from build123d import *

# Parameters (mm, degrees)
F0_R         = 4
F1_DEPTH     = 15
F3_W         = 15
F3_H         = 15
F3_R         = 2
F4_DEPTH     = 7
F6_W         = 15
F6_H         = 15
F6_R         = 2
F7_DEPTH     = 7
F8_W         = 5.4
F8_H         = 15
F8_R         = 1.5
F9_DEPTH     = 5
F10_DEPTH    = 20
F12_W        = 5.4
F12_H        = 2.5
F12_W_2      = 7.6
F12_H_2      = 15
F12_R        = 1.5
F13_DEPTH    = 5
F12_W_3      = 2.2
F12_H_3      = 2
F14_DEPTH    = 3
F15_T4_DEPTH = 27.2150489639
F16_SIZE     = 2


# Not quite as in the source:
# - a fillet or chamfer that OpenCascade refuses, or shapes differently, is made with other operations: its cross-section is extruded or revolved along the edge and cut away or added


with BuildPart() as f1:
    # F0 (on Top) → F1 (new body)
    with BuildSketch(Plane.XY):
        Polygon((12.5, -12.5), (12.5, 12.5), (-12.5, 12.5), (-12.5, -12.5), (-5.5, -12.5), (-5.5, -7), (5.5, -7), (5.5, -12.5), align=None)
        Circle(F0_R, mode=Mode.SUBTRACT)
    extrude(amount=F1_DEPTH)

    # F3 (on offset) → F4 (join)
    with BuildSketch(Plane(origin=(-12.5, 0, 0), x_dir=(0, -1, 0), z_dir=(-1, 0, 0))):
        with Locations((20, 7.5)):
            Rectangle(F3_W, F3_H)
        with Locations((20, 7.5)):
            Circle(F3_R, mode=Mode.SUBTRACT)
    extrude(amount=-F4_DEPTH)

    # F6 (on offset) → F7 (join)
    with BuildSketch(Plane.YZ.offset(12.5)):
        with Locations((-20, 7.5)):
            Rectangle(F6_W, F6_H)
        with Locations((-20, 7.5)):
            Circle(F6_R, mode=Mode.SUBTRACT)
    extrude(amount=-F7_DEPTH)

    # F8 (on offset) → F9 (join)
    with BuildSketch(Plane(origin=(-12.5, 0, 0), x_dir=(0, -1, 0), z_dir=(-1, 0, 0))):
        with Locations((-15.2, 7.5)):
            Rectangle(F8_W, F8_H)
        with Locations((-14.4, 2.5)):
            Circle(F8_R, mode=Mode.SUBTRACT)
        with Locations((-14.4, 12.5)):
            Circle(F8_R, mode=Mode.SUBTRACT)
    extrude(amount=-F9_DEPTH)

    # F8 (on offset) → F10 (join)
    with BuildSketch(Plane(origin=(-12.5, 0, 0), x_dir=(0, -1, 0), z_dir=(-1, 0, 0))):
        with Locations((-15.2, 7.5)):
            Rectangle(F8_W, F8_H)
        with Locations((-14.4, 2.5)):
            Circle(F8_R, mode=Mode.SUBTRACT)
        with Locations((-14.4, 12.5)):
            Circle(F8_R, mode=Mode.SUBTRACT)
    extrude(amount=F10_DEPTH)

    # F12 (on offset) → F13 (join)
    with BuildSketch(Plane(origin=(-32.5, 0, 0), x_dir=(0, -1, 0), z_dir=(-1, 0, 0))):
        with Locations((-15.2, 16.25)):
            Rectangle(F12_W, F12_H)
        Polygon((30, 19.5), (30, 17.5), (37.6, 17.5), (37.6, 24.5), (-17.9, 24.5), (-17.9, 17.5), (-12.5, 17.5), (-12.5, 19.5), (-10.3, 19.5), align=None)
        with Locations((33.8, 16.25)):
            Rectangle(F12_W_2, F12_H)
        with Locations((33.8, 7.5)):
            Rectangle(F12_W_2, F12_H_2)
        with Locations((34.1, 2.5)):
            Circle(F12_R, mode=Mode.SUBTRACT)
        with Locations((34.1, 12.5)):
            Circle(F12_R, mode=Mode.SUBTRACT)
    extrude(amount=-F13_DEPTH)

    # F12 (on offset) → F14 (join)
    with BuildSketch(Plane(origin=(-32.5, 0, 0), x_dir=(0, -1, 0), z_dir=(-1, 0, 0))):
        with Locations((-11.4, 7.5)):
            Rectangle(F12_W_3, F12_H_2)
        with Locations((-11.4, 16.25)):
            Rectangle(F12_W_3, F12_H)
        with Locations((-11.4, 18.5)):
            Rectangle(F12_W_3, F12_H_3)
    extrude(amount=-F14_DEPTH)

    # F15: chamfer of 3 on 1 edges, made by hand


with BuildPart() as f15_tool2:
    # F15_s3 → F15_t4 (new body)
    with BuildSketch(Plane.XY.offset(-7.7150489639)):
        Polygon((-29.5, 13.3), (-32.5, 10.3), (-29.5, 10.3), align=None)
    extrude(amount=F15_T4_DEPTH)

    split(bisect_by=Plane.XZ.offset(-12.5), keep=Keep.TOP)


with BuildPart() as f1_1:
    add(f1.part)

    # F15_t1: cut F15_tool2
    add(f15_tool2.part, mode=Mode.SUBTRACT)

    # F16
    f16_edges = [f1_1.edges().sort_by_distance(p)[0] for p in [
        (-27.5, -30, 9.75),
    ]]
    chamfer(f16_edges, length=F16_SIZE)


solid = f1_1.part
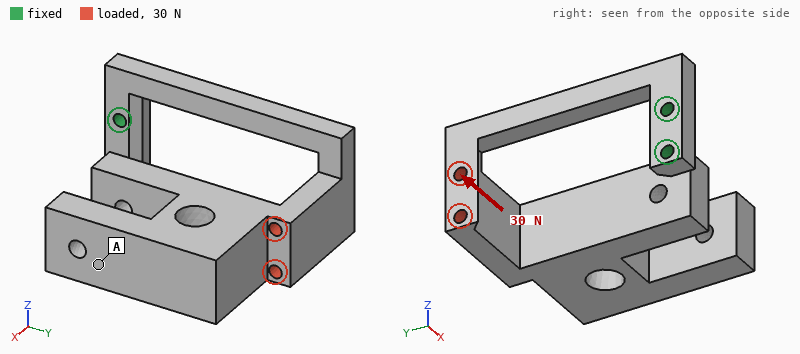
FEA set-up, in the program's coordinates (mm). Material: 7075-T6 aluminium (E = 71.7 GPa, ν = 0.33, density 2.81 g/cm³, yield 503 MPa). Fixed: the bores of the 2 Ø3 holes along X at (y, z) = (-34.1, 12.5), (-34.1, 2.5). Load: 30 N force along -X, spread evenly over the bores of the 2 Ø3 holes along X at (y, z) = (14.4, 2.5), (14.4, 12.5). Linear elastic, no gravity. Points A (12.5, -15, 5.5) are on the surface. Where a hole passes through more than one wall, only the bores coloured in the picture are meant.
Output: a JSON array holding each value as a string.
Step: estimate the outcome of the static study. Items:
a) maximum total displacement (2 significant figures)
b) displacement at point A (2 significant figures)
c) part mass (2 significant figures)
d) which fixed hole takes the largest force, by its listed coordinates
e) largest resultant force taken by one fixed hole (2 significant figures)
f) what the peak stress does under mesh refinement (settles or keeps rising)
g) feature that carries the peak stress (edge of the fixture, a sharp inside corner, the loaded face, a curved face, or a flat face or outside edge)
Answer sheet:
["0.82 mm", "0.64 mm", "41 g", "(-34.1, 12.5)", "30 N", "keeps rising", "edge of the fixture"]
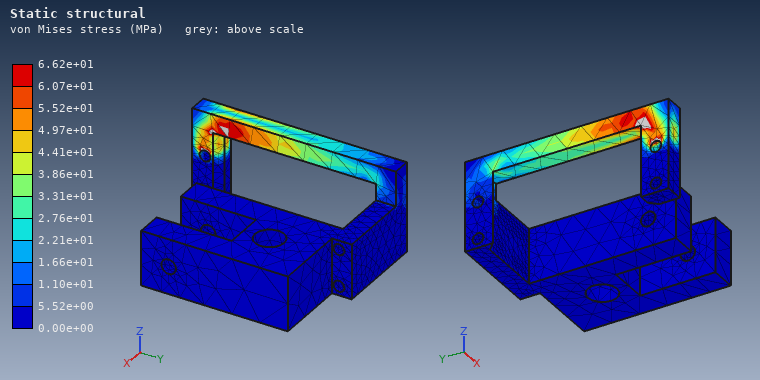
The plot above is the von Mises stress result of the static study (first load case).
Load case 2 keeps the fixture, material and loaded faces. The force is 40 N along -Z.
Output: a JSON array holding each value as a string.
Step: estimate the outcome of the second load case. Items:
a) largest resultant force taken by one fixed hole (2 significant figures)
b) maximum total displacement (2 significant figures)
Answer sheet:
["69 N", "0.89 mm"]
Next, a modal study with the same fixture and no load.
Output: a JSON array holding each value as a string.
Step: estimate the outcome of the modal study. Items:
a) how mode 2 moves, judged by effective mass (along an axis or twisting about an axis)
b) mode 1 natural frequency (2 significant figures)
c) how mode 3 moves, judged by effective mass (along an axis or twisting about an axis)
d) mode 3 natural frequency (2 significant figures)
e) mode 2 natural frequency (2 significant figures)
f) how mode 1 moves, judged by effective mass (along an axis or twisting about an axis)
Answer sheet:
["along Y", "160 Hz", "along X", "350 Hz", "180 Hz", "along Z"]
